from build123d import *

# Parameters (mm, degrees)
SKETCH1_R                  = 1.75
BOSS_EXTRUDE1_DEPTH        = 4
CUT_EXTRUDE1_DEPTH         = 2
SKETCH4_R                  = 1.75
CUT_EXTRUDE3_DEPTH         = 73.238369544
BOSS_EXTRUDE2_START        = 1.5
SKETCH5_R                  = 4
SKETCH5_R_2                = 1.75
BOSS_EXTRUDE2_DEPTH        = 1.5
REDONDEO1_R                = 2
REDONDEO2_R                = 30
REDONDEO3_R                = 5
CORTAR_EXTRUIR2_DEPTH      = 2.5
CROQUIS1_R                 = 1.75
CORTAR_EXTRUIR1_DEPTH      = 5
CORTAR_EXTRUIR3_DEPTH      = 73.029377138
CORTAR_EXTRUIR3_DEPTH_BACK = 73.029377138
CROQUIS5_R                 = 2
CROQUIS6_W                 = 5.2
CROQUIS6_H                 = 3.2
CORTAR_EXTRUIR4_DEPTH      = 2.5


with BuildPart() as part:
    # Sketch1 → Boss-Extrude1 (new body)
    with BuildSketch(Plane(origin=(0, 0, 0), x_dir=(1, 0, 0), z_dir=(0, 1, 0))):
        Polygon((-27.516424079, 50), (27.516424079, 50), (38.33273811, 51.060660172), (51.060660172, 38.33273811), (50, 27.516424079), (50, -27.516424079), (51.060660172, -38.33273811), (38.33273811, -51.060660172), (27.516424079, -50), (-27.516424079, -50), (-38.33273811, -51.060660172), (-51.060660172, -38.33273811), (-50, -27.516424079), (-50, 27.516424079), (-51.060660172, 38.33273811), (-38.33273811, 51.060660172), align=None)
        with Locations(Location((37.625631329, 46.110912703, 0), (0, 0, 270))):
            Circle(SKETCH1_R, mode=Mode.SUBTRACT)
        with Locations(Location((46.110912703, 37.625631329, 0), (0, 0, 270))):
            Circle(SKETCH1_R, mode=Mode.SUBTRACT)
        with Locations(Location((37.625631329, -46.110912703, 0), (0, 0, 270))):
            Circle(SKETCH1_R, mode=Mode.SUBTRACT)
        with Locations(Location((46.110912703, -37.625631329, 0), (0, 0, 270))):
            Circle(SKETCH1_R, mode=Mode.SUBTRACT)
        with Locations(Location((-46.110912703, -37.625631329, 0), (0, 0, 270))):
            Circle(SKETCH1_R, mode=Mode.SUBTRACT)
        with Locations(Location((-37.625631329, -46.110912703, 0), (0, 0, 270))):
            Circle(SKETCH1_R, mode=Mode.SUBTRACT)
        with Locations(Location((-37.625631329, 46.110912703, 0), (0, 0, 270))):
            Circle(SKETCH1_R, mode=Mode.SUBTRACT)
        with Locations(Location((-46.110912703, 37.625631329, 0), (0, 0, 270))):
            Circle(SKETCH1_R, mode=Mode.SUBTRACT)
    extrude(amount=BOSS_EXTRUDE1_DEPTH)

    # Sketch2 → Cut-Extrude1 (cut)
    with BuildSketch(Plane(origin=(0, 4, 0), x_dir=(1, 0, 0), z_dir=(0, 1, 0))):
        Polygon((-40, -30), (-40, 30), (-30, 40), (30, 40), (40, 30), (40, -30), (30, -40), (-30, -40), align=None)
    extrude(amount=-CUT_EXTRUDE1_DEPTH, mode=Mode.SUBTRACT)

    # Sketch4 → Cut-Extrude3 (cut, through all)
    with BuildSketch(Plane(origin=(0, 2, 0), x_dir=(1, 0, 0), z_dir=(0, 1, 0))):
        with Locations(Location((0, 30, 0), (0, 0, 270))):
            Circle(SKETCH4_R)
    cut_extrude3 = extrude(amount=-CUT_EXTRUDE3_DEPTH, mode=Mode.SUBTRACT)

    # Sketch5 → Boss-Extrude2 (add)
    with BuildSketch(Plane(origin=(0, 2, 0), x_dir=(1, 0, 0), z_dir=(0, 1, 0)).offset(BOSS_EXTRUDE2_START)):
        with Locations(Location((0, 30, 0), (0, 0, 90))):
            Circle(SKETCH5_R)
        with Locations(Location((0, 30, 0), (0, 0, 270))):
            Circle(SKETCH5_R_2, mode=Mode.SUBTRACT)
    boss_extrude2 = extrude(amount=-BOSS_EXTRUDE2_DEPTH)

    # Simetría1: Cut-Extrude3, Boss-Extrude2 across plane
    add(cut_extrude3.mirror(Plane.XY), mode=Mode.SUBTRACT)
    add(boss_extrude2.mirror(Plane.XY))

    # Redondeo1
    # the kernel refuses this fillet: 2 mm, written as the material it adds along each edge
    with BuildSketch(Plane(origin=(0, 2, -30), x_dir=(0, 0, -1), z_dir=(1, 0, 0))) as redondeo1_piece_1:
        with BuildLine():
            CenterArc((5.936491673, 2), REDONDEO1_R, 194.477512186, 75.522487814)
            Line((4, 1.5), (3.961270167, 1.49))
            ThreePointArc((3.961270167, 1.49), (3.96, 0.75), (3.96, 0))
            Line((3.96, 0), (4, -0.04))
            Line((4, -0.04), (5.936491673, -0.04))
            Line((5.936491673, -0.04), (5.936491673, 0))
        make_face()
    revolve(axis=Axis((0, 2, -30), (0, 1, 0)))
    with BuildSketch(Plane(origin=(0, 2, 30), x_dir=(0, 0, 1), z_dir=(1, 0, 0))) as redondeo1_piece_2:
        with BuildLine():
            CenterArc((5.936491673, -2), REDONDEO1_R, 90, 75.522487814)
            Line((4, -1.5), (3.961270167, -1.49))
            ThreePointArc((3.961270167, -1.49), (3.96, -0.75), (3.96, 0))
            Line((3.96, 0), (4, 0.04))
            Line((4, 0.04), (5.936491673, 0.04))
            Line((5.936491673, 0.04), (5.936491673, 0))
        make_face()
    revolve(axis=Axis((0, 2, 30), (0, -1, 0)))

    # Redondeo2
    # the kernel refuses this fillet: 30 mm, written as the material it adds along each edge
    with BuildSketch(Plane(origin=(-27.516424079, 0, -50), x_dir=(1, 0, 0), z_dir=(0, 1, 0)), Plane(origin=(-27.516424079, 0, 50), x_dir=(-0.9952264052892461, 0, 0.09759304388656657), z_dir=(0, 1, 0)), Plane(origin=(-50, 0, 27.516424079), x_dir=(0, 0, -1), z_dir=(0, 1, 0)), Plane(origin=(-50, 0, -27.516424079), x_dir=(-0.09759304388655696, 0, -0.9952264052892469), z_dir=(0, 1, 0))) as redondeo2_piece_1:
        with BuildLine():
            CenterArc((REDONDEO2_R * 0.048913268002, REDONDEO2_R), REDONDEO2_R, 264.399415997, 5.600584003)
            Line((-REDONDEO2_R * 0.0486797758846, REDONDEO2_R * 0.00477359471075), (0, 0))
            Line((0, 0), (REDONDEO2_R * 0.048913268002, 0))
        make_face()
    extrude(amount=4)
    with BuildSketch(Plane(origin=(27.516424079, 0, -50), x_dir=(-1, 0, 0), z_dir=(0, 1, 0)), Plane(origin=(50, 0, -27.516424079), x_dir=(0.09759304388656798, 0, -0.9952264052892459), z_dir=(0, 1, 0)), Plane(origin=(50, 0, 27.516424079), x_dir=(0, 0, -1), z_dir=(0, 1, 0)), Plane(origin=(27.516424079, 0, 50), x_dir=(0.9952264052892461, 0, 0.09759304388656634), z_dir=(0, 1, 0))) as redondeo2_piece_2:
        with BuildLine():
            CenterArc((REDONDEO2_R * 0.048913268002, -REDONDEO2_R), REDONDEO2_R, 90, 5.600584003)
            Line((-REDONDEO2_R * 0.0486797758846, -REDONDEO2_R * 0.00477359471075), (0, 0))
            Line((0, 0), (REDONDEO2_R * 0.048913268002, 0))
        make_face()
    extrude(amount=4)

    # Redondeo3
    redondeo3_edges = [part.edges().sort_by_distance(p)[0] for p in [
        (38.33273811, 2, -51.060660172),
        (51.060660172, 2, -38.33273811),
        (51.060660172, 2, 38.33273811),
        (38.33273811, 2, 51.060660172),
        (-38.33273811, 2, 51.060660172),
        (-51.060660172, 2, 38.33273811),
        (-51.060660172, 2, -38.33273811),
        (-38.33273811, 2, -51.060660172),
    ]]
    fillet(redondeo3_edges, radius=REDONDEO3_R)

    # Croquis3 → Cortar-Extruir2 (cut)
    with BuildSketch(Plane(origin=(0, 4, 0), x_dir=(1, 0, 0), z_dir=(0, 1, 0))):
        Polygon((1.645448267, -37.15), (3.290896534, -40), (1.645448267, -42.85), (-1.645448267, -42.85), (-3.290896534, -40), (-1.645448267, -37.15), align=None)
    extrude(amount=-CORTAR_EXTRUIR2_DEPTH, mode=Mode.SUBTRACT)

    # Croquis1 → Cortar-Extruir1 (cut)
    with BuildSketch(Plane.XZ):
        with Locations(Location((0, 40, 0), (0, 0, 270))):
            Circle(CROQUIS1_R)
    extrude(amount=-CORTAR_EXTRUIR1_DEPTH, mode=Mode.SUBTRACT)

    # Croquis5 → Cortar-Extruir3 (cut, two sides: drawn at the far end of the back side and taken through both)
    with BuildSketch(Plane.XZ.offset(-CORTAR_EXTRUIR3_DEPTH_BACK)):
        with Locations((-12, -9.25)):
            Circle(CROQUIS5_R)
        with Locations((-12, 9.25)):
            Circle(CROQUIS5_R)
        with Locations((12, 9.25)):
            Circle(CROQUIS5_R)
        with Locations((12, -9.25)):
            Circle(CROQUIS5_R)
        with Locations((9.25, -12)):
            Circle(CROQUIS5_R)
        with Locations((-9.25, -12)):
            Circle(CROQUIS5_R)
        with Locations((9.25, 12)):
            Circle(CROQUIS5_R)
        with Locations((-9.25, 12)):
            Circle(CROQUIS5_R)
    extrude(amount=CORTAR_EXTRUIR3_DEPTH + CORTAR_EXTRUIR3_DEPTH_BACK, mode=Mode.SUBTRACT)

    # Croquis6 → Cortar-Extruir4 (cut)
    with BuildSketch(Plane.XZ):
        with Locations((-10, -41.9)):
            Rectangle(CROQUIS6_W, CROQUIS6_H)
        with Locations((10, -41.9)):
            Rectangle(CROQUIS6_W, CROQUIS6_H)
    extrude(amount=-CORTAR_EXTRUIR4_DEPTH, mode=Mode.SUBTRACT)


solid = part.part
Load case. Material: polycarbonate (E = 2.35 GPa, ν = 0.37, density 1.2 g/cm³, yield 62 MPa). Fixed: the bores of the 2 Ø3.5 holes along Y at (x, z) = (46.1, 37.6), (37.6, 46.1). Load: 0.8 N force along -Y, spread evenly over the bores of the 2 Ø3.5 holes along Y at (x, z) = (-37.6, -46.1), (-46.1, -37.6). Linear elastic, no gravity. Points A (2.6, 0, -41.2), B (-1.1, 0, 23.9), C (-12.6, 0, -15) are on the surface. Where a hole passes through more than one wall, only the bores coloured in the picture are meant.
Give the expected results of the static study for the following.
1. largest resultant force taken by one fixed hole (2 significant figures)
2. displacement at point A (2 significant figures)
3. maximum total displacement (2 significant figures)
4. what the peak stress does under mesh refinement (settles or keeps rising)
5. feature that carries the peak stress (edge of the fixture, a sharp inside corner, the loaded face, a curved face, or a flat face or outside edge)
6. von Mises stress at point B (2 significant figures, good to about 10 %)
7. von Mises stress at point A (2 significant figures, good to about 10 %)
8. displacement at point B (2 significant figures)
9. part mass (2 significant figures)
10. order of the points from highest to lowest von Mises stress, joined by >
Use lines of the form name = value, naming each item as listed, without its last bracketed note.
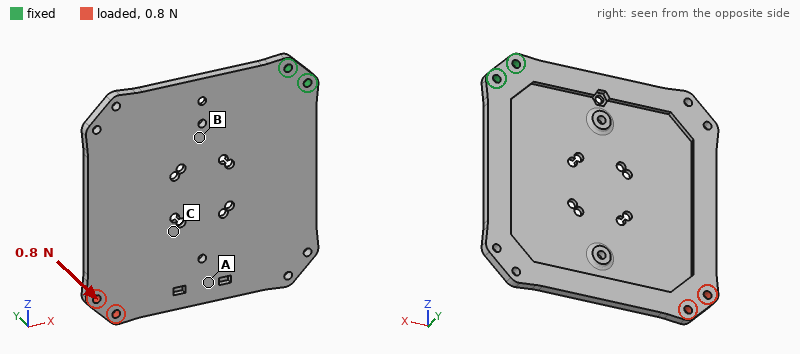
largest resultant force taken by one fixed hole = 3.7 N
displacement at point A = 0.82 mm
maximum total displacement = 1.4 mm
what the peak stress does under mesh refinement = keeps rising
feature that carries the peak stress = edge of the fixture
von Mises stress at point B = 0.50 MPa
von Mises stress at point A = 0.30 MPa
displacement at point B = 0.25 mm
part mass = 32 g
order of the points from highest to lowest von Mises stress, joined by > = B > A > C
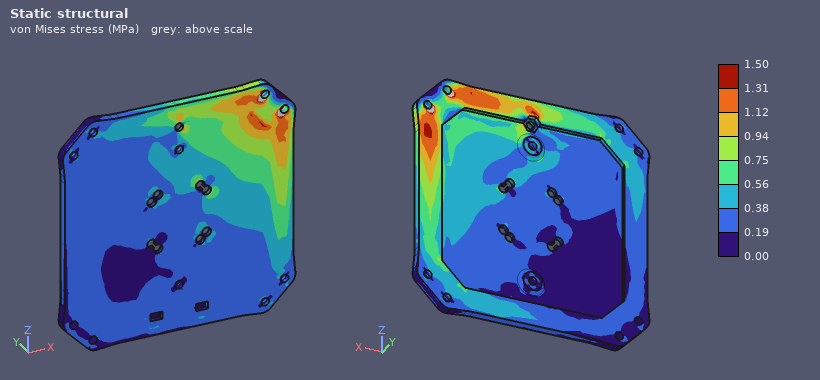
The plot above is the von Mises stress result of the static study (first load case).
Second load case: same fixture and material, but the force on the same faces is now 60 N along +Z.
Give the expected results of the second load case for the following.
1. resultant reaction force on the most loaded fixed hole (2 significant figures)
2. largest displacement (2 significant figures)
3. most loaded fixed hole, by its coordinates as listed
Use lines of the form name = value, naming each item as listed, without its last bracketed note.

resultant reaction force on the most loaded fixed hole = 350 N
largest displacement = 1.5 mm
most loaded fixed hole, by its coordinates as listed = (37.6, 46.1)
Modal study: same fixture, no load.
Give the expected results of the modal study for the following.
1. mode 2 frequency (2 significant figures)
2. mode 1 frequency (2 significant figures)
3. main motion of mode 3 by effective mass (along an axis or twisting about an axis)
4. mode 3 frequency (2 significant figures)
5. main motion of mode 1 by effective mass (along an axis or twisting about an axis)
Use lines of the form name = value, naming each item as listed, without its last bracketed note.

mode 2 frequency = 95 Hz
mode 1 frequency = 46 Hz
main motion of mode 3 by effective mass = along Y
mode 3 frequency = 210 Hz
main motion of mode 1 by effective mass = along Y
